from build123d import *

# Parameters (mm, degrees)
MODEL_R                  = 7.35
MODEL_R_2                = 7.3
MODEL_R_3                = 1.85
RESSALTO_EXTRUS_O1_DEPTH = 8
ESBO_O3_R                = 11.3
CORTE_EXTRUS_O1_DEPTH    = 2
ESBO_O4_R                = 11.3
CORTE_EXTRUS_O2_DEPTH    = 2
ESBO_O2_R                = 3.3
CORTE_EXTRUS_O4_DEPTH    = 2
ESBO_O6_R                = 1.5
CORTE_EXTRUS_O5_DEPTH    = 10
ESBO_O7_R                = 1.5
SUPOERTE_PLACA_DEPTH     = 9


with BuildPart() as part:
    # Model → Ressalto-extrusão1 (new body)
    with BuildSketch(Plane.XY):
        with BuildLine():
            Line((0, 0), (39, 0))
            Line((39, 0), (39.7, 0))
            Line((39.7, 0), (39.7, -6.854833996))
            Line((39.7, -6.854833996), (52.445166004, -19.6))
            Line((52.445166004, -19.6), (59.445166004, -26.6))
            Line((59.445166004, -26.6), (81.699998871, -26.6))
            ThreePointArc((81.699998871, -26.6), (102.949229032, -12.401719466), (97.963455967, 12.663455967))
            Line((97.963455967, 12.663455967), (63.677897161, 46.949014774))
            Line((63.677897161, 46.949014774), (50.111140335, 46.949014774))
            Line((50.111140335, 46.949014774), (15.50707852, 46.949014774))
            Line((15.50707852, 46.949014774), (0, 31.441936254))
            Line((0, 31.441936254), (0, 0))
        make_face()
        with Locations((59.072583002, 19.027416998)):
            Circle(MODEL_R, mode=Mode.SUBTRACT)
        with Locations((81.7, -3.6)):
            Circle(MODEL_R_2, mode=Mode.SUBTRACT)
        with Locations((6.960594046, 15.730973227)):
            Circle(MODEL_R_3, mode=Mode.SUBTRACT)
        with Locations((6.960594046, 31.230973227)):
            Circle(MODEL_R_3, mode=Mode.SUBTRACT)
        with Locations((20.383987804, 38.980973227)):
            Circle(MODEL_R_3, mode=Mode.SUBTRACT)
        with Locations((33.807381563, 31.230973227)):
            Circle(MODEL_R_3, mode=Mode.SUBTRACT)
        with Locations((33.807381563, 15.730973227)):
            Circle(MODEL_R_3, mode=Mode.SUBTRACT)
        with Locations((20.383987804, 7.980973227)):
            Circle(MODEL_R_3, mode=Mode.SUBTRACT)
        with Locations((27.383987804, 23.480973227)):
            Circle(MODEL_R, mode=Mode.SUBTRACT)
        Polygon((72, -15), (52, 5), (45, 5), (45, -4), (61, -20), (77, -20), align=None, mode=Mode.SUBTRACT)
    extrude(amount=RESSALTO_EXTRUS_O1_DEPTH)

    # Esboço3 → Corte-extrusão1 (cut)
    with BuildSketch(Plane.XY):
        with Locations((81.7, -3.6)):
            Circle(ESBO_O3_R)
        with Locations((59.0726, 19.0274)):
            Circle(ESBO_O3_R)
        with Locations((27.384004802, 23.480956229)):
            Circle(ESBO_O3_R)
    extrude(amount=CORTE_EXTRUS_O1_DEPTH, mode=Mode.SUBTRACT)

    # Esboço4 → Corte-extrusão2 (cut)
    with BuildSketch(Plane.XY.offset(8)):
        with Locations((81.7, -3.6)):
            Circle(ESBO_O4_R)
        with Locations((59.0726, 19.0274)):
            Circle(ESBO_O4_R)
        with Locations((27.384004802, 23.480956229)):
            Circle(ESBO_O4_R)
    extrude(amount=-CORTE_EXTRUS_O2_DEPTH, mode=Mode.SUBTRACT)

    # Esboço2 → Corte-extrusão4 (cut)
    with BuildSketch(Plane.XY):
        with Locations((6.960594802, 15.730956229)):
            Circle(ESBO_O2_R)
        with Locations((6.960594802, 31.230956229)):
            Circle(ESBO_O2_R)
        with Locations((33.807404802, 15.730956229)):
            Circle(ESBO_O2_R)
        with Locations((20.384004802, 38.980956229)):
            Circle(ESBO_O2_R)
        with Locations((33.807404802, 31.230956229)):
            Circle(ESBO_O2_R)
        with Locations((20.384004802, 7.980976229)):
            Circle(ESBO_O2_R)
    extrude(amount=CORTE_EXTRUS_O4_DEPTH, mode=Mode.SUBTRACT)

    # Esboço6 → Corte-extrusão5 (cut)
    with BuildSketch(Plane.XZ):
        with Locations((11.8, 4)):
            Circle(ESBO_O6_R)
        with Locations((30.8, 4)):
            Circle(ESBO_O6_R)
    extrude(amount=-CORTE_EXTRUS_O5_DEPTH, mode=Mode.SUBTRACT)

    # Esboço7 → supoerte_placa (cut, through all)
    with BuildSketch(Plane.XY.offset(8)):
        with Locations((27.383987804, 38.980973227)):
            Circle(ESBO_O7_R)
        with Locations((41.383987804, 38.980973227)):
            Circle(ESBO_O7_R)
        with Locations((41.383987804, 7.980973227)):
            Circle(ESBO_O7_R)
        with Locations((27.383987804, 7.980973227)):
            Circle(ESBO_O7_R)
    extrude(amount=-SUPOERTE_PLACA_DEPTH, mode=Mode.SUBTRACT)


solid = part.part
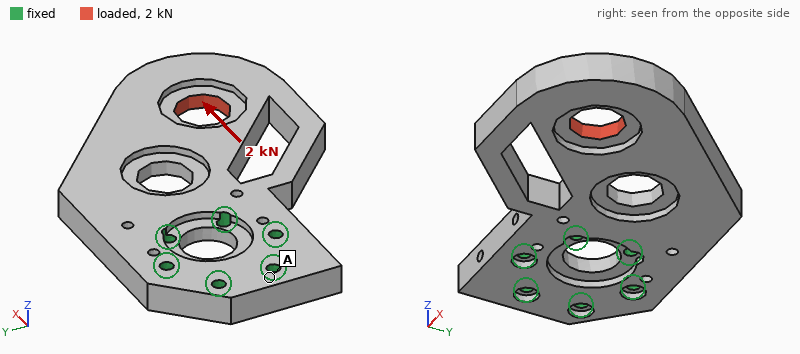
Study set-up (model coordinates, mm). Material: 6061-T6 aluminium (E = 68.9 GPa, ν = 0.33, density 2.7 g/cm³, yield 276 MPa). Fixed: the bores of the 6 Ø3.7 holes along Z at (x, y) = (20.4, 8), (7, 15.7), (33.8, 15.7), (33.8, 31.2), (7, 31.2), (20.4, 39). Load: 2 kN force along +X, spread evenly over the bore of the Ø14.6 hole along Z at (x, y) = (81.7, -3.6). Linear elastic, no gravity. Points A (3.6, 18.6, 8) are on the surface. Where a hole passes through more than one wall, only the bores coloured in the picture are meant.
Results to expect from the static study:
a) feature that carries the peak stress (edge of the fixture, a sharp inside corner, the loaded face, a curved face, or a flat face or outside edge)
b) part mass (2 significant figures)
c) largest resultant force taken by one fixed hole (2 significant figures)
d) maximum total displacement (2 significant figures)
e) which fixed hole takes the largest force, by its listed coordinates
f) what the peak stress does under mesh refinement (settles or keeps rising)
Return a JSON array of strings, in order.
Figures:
["edge of the fixture", "87 g", "1.7 kN", "69 µm", "(33.8, 15.7)", "keeps rising"]
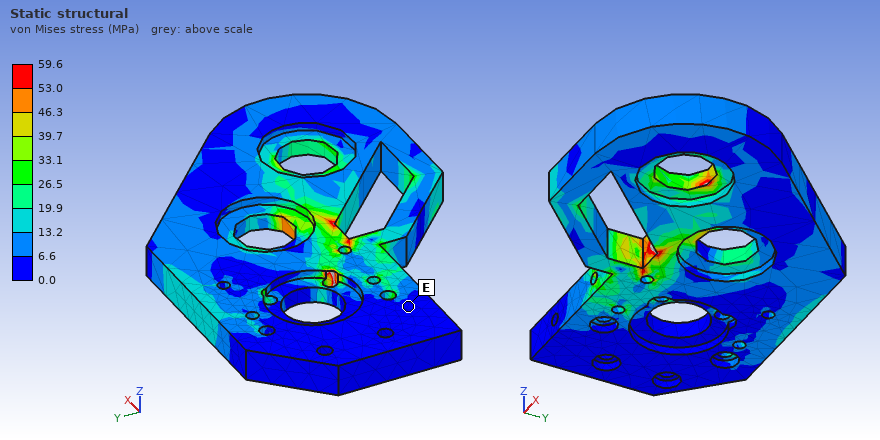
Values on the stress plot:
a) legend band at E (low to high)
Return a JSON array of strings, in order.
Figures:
["0.0 to 6.6 MPa"]
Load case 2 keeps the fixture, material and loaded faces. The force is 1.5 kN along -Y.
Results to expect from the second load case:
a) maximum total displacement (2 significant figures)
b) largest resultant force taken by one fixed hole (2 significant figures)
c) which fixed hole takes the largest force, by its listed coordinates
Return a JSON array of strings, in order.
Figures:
["75 µm", "1.7 kN", "(33.8, 15.7)"]
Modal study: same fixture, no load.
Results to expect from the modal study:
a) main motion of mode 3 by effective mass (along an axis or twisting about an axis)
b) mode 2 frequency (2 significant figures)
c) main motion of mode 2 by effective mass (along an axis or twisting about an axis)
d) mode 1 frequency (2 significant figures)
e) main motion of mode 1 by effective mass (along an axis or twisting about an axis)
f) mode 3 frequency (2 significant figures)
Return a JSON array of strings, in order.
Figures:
["along Y", "2700 Hz", "twisting about X", "990 Hz", "along Z", "3900 Hz"]
